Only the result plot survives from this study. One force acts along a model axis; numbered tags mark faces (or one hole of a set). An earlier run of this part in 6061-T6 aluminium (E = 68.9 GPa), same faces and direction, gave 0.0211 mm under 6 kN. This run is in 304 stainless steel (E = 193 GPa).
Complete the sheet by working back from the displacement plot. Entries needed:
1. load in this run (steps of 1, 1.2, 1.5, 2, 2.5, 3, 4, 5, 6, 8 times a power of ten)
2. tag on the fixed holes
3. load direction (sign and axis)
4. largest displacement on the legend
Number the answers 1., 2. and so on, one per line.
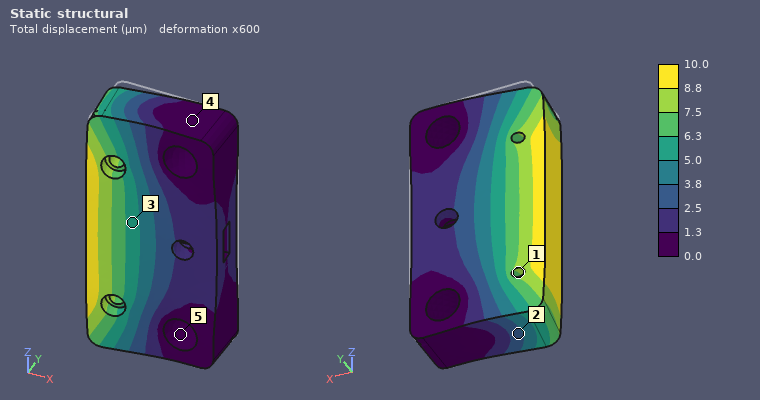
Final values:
1. 8 kN
2. 5
3. -Y
4. 10.0 µm
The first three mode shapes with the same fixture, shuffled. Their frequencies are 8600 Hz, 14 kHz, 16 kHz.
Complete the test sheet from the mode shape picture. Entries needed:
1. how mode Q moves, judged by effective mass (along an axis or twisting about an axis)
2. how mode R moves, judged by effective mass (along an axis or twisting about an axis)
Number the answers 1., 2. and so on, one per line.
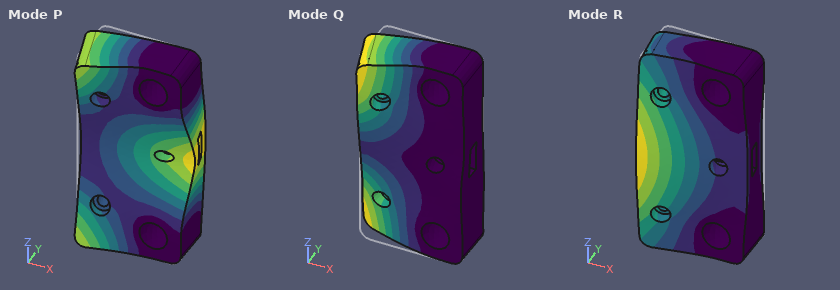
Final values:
1. twisting about X
2. along Y
